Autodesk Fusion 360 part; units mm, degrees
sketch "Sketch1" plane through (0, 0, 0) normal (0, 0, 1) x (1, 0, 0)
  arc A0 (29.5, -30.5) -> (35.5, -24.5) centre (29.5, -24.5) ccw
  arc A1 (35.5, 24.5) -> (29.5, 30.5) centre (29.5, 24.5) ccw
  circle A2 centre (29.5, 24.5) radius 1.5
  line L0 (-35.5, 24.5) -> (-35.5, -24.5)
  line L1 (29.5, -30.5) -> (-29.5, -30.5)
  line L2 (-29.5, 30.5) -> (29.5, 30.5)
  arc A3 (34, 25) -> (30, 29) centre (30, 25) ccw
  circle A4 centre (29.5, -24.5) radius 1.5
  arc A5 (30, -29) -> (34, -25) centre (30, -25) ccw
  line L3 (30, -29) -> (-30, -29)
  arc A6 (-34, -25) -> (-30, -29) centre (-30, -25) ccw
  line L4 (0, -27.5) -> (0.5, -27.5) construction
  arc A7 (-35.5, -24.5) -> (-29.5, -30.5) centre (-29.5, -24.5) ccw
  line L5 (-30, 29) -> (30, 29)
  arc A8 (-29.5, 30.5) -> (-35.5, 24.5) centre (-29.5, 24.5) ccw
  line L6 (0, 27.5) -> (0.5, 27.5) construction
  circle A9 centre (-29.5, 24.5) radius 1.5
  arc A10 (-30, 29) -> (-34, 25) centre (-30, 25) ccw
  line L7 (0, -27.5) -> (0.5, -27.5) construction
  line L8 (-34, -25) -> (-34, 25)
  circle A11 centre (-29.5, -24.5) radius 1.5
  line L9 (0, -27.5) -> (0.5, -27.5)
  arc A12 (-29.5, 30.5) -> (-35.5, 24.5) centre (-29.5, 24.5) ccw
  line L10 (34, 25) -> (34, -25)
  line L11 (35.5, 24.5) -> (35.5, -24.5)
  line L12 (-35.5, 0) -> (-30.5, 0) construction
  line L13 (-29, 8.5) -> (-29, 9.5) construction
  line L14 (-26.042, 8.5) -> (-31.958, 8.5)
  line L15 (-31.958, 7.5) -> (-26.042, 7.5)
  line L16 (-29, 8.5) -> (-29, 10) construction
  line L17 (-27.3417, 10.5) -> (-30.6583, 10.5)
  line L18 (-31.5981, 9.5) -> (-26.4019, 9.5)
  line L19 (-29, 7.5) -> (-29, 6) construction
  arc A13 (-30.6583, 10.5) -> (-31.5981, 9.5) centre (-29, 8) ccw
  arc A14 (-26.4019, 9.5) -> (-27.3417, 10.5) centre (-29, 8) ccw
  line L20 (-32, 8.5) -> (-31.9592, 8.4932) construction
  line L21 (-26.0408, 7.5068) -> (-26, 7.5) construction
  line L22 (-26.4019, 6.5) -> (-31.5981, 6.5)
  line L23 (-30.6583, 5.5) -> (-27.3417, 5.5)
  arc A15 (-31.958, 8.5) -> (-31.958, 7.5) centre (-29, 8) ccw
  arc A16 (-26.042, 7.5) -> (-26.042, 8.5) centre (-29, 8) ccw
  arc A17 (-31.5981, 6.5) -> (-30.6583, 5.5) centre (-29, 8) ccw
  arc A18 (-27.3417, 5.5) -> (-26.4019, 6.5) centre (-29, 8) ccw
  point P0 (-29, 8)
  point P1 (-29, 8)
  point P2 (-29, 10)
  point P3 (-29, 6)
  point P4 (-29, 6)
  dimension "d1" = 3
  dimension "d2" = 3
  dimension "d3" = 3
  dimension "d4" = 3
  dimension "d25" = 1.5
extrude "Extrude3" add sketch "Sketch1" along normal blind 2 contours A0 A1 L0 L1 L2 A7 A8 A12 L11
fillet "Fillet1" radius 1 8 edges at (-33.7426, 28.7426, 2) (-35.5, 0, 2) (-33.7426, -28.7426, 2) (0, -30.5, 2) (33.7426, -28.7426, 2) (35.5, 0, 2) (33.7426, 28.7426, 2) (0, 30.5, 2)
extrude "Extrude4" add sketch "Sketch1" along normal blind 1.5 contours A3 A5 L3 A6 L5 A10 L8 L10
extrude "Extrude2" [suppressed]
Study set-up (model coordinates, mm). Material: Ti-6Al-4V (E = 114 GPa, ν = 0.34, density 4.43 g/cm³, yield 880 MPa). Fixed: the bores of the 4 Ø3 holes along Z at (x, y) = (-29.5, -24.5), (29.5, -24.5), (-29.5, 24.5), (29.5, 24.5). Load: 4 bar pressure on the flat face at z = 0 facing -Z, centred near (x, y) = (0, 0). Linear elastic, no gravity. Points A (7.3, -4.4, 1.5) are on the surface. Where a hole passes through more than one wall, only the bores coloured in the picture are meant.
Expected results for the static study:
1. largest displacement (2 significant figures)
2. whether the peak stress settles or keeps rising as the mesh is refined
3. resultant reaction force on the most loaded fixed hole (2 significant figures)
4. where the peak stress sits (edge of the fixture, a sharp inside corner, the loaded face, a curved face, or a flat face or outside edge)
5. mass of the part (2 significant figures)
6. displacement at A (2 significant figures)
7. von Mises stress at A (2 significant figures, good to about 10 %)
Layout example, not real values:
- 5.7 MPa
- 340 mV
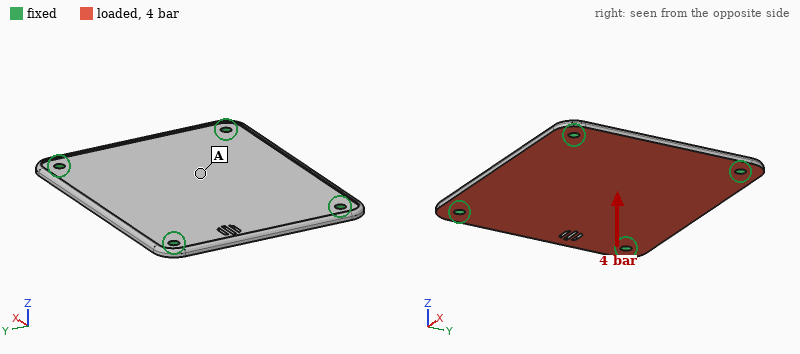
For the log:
- 0.67 mm
- keeps rising
- 430 N
- edge of the fixture
- 29 g
- 0.62 mm
- 150 MPa
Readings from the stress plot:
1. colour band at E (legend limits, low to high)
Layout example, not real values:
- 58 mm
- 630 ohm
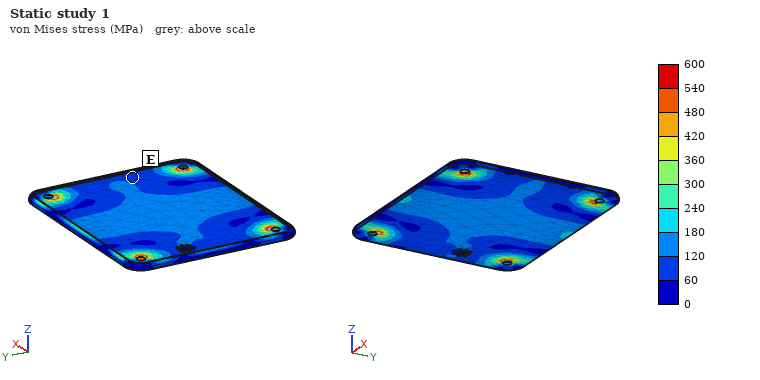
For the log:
- 60 to 120 MPa
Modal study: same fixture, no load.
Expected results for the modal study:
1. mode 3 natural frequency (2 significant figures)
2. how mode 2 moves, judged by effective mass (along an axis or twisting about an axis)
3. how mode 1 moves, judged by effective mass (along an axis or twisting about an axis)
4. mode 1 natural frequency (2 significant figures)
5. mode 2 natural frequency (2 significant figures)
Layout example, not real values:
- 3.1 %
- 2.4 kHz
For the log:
- 3400 Hz
- twisting about X
- along Z
- 1800 Hz
- 2800 Hz
